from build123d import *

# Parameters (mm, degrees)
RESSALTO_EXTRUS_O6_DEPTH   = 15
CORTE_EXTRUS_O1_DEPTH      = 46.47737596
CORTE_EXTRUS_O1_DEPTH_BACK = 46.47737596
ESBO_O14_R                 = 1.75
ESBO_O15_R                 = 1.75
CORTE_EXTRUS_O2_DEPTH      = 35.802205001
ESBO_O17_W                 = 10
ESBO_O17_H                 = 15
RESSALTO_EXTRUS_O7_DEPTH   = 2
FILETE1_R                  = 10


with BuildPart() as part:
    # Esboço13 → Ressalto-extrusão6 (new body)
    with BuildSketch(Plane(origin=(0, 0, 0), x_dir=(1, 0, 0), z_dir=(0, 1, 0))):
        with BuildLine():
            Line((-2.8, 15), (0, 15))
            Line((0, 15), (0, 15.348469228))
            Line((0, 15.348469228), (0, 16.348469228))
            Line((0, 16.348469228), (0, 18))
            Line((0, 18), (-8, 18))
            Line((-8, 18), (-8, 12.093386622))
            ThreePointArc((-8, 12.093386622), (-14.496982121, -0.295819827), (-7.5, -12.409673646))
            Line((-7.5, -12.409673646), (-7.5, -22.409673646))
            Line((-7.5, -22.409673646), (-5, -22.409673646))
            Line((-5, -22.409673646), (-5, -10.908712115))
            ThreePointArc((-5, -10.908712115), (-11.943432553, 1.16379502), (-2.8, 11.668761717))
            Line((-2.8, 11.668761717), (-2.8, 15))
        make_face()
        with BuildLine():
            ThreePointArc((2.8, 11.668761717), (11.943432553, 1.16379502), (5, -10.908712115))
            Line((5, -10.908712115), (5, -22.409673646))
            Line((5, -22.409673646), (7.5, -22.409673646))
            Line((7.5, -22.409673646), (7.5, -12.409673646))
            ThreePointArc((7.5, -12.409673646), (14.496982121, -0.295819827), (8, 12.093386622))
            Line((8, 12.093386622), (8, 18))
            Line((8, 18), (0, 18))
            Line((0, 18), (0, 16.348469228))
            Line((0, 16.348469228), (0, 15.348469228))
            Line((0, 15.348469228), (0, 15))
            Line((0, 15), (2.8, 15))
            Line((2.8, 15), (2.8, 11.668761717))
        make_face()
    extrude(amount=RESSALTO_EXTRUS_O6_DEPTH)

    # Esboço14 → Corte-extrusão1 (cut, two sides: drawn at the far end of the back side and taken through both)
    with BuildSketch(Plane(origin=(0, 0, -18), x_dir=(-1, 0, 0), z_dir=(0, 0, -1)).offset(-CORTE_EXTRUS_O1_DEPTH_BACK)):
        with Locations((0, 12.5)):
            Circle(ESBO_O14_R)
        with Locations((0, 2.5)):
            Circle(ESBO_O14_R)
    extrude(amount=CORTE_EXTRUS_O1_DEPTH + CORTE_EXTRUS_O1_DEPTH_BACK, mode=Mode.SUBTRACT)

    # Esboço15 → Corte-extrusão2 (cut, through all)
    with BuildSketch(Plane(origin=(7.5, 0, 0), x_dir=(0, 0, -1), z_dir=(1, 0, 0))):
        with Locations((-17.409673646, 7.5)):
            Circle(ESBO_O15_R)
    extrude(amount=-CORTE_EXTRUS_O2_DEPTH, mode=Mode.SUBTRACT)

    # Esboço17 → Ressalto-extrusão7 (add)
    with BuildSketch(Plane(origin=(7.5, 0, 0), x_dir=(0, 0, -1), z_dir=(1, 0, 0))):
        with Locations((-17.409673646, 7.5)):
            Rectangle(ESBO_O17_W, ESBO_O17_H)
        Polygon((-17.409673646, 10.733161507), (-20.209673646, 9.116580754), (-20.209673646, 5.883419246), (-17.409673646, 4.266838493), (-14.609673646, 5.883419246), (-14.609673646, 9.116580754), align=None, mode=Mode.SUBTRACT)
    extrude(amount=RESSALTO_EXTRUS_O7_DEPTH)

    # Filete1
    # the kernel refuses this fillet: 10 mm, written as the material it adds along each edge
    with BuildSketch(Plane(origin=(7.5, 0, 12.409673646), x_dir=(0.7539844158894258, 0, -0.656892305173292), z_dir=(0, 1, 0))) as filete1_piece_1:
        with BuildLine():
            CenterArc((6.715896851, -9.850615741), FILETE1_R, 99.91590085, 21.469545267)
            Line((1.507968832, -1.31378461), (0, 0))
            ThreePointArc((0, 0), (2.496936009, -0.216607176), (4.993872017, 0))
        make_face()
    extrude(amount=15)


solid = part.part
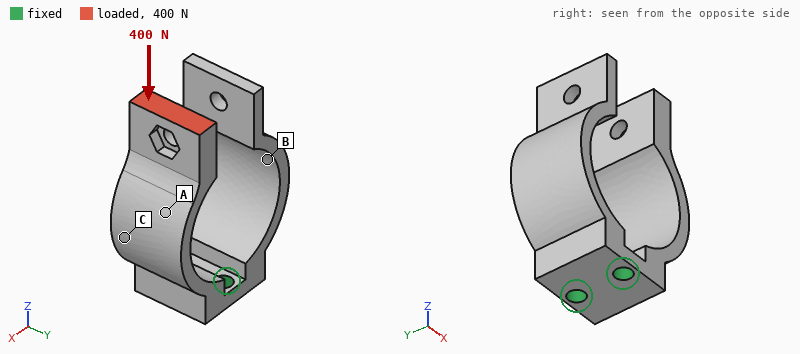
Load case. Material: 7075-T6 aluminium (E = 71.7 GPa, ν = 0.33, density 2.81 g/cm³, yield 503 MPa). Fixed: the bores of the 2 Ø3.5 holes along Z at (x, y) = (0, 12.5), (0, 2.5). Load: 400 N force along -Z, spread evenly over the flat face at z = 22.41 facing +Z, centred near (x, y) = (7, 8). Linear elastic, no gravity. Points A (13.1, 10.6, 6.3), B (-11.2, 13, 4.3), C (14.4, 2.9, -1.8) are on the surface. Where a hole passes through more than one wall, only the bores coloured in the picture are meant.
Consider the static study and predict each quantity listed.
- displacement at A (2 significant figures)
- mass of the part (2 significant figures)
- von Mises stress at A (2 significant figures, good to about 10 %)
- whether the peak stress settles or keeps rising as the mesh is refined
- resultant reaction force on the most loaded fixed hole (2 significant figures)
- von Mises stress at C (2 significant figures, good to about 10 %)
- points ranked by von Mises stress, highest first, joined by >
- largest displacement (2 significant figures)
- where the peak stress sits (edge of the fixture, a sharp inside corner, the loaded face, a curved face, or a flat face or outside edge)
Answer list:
0.12 mm
12 g
93 MPa
keeps rising
200 N
120 MPa
C > A > B
0.56 mm
edge of the fixture
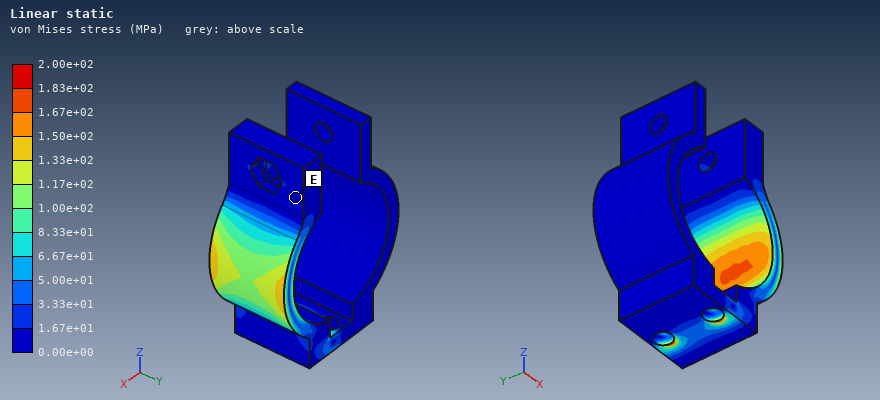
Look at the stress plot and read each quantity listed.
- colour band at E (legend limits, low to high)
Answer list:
0.00e+00 to 1.67e+01 MPa
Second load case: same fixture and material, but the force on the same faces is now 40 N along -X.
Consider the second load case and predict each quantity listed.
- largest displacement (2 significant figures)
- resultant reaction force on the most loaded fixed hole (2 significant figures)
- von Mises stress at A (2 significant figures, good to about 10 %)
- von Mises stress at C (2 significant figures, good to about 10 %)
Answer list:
0.53 mm
27 N
37 MPa
55 MPa
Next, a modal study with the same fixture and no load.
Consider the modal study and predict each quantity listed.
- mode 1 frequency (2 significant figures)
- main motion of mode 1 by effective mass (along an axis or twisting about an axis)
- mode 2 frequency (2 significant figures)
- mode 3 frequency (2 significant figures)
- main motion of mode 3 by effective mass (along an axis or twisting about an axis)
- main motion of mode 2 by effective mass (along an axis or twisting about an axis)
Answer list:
1100 Hz
along X
1400 Hz
2300 Hz
along Y
along X
